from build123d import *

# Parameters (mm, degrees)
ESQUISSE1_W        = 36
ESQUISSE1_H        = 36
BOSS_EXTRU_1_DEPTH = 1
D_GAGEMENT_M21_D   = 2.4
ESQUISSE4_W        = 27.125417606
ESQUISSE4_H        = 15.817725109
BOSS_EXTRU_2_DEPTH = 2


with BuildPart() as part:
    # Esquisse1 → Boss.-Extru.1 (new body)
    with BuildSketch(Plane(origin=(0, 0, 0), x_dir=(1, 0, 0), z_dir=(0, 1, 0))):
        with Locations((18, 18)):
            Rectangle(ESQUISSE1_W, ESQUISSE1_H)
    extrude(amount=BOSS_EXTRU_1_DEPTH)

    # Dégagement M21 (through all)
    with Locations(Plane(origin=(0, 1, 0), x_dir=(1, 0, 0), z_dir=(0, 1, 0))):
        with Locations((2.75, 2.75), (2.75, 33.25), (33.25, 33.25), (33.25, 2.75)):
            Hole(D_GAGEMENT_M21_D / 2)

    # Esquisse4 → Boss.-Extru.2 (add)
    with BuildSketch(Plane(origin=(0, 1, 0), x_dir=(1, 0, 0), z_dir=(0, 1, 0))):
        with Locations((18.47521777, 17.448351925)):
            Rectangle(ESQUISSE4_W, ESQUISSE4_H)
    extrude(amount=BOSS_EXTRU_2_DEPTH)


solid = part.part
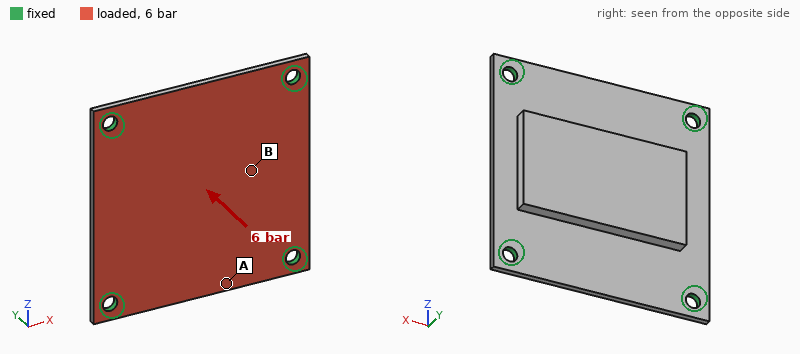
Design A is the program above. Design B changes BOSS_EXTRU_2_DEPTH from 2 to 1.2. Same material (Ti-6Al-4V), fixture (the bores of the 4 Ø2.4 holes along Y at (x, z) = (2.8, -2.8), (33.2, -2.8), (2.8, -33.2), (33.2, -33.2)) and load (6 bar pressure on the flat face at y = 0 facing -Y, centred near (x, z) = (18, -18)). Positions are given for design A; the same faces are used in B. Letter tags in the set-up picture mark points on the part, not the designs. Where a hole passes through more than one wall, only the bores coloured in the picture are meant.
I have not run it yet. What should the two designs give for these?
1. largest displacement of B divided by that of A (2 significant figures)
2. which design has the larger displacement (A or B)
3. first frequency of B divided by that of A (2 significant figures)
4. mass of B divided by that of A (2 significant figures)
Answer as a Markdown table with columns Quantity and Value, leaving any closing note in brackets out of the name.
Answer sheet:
| Quantity | Value |
|---|---|
| largest displacement of B divided by that of A | 1.2 |
| which design has the larger displacement | B |
| first frequency of B divided by that of A | 1.00 |
| mass of B divided by that of A | 0.84 |
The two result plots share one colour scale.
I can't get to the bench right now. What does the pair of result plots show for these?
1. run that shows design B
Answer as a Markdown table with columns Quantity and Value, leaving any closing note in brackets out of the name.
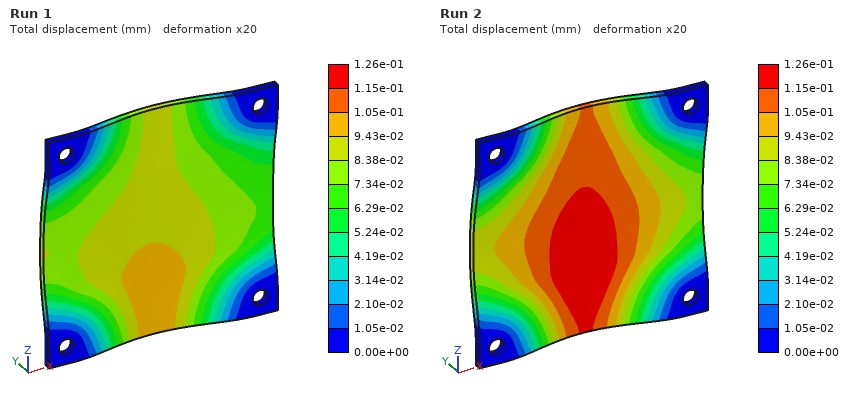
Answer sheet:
| Quantity | Value |
|---|---|
| run that shows design B | Run 2 |
